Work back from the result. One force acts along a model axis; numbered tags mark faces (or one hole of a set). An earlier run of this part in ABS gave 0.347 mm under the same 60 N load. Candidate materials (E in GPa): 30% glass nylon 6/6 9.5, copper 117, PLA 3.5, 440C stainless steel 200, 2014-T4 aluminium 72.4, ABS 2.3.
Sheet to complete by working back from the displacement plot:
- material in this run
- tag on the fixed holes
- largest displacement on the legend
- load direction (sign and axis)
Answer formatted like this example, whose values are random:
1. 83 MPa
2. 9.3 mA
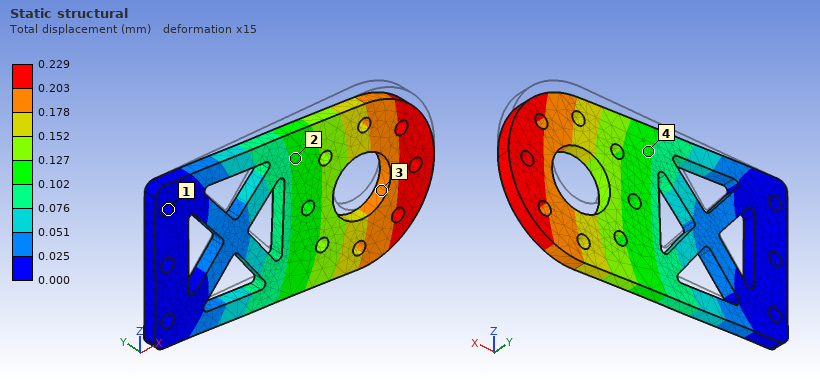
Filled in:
1. PLA
2. 1
3. 0.229 mm
4. -Z
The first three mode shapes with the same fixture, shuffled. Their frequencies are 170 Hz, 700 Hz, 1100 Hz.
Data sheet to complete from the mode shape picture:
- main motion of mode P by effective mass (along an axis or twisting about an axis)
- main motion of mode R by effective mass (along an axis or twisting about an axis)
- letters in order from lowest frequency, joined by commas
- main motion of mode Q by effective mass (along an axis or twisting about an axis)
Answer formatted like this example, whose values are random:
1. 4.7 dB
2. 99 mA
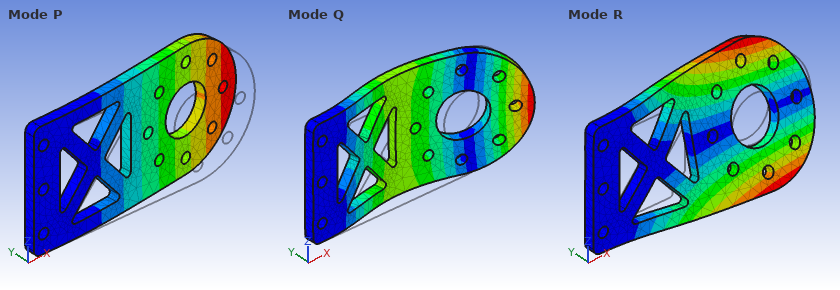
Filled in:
1. along Y
2. twisting about X
3. P, R, Q
4. along Y
